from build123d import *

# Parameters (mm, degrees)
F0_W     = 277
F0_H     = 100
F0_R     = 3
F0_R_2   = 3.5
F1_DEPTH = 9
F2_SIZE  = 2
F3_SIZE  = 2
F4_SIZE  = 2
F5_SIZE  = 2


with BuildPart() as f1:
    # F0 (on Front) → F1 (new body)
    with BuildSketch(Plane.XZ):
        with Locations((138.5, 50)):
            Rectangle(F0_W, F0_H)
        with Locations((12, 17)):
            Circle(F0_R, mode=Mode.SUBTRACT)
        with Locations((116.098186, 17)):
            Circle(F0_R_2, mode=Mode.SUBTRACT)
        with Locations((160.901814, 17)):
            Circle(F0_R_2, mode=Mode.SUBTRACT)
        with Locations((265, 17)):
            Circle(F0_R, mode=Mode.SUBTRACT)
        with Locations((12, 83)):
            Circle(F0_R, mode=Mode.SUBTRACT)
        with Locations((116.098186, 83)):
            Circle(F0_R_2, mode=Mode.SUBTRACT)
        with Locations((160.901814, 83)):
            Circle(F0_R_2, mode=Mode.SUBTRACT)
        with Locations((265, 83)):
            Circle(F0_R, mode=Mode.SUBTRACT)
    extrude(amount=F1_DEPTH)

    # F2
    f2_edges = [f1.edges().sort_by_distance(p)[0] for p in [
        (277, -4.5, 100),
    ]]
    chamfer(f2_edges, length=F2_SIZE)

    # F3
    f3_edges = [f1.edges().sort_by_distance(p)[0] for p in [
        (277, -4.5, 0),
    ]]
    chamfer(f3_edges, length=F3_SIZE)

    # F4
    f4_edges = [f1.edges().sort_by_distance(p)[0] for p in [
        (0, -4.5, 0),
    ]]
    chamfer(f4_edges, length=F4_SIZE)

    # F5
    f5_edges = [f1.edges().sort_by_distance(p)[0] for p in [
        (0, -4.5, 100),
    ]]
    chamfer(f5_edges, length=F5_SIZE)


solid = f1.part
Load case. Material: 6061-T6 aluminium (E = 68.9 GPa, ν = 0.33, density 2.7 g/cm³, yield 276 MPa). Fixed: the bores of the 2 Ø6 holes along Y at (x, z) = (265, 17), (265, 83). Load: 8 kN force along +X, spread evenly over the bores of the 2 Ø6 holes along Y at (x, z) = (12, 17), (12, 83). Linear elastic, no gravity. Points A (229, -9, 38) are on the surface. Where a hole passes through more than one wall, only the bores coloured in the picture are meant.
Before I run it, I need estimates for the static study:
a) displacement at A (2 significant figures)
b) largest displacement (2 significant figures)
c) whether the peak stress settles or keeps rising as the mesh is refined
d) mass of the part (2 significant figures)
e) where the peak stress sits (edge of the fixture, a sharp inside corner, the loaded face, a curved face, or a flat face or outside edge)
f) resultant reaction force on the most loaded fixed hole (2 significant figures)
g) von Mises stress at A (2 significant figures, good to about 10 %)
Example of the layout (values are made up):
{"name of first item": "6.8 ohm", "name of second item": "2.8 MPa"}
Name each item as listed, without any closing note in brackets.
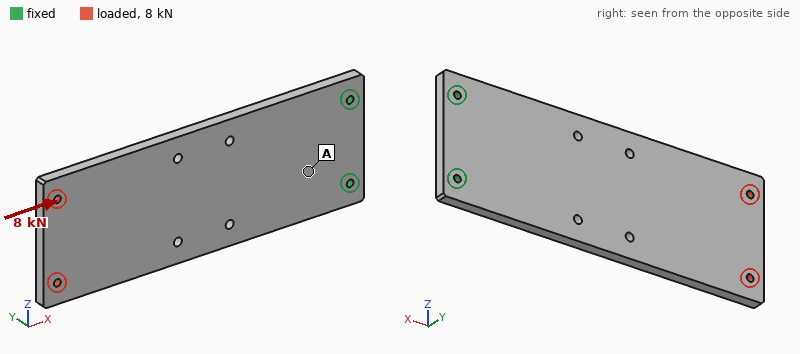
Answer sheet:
{"displacement at A": "8.0 µm", "largest displacement": "41 µm", "whether the peak stress settles or keeps rising as the mesh is refined": "keeps rising", "mass of the part": "670 g", "where the peak stress sits": "edge of the fixture", "resultant reaction force on the most loaded fixed hole": "4.0 kN", "von Mises stress at A": "7.7 MPa"}
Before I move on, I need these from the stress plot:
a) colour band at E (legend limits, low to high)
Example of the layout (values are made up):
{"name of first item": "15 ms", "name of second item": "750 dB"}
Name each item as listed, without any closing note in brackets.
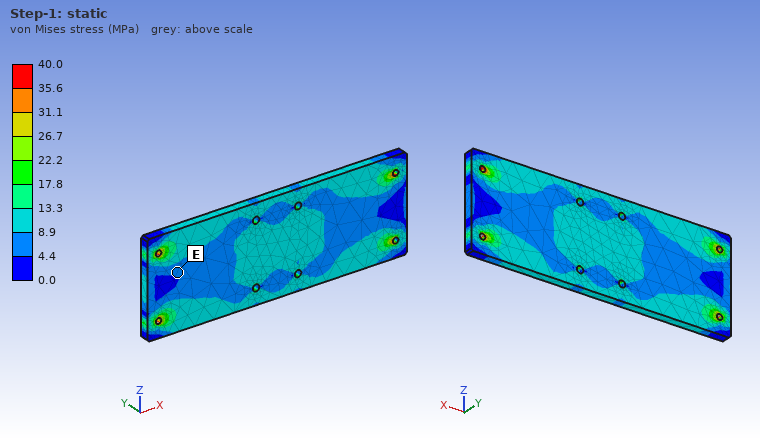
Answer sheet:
{"colour band at E": "4.4 to 8.9 MPa"}
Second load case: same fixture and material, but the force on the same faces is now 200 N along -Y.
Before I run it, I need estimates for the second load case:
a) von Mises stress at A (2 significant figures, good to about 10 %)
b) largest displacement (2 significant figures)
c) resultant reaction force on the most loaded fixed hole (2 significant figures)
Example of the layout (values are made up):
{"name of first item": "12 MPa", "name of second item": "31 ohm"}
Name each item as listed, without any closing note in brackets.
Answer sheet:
{"von Mises stress at A": "30 MPa", "largest displacement": "3.0 mm", "resultant reaction force on the most loaded fixed hole": "100 N"}
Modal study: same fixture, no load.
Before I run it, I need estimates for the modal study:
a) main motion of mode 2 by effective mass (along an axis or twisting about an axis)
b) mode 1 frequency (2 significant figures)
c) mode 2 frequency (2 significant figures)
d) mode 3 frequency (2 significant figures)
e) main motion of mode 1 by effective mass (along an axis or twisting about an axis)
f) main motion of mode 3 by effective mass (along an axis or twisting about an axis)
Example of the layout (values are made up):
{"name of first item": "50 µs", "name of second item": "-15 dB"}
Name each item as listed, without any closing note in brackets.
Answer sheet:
{"main motion of mode 2 by effective mass": "twisting about X", "mode 1 frequency": "100 Hz", "mode 2 frequency": "560 Hz", "mode 3 frequency": "630 Hz", "main motion of mode 1 by effective mass": "along Y", "main motion of mode 3 by effective mass": "along Y"}
